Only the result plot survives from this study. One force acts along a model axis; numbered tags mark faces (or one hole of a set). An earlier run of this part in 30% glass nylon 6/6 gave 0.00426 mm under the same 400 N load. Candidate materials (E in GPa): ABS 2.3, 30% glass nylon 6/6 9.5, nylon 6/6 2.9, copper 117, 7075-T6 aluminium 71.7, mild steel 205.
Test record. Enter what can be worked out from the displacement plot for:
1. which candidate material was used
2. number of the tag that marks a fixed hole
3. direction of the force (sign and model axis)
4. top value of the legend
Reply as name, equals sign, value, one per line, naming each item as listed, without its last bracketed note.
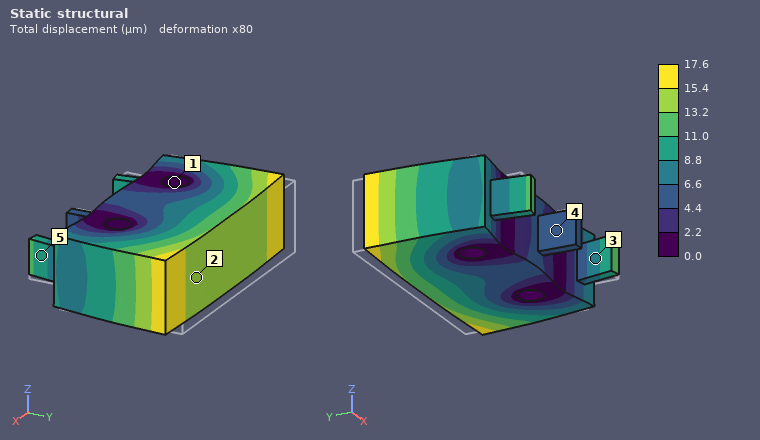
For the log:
which candidate material was used = ABS
number of the tag that marks a fixed hole = 1
direction of the force = -Y
top value of the legend = 17.6 µm
